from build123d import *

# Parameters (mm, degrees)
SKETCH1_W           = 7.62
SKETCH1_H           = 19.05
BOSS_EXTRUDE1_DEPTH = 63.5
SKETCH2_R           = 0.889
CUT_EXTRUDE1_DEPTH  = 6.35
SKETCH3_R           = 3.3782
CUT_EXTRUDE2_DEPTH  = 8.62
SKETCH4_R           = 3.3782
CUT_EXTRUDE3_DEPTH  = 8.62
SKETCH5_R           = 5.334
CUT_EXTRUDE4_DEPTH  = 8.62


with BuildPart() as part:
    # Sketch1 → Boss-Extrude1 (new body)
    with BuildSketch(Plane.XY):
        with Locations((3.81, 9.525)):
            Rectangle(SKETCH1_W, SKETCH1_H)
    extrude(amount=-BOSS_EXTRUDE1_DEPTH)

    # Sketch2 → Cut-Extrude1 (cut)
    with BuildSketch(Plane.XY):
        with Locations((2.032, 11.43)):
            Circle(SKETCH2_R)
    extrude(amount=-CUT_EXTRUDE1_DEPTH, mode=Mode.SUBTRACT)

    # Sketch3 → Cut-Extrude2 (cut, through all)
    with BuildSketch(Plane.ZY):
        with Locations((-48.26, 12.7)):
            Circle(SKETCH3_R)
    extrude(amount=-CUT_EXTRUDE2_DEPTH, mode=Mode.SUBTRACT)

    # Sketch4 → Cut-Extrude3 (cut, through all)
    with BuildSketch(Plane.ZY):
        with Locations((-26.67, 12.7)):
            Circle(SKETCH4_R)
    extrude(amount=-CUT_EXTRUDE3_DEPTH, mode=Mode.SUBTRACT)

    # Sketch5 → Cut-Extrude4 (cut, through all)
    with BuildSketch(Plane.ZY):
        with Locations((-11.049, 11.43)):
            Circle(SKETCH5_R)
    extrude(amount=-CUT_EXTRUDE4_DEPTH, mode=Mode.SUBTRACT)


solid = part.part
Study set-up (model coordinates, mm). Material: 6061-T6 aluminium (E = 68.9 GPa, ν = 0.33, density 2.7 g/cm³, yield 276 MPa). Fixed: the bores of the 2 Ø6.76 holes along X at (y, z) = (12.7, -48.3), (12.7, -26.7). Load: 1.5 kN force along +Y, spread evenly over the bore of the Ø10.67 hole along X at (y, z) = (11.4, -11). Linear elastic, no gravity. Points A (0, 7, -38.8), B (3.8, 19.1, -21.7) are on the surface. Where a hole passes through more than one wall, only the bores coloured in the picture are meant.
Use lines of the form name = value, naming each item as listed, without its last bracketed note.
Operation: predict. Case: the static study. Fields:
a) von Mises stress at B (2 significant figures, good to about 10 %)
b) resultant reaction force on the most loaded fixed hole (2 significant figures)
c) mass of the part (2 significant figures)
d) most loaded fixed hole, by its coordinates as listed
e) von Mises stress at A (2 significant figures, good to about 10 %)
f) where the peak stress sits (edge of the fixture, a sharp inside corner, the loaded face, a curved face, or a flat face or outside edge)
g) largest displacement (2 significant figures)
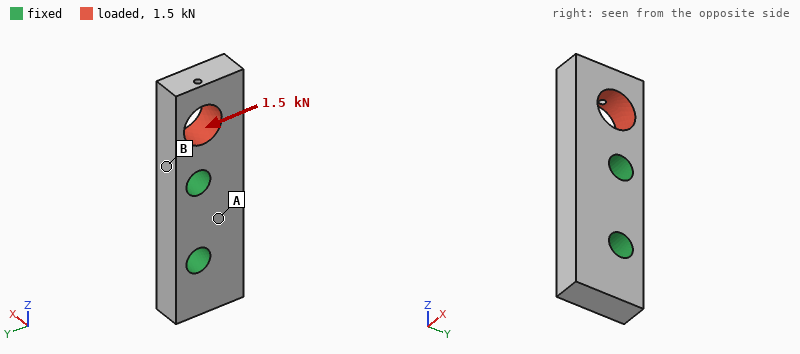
von Mises stress at B = 47 MPa
resultant reaction force on the most loaded fixed hole = 2.0 kN
mass of the part = 22 g
most loaded fixed hole, by its coordinates as listed = (12.7, -26.7)
von Mises stress at A = 11 MPa
where the peak stress sits = edge of the fixture
largest displacement = 46 µm
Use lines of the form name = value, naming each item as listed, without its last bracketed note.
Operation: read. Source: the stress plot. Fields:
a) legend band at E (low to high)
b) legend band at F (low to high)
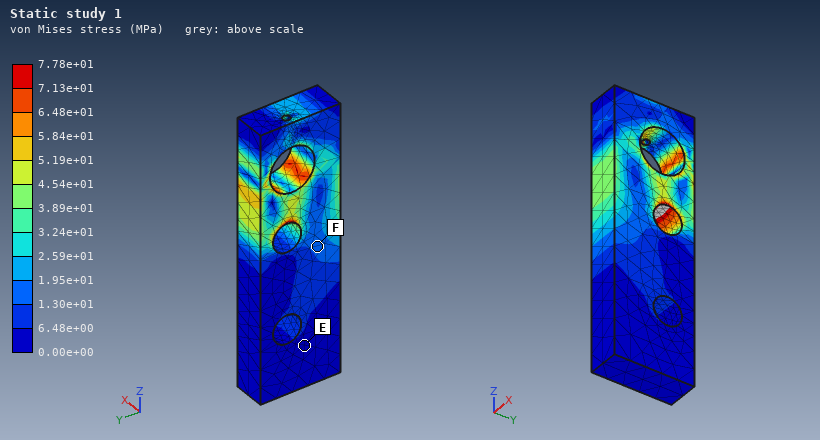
legend band at E = 0.00e+00 to 6.48e+00 MPa
legend band at F = 1.30e+01 to 1.95e+01 MPa
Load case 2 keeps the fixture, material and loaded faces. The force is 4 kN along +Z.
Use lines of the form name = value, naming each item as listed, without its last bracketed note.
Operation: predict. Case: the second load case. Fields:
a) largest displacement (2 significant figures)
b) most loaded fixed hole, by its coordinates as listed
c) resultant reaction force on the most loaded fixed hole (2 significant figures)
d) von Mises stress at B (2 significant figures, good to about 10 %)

largest displacement = 20 µm
most loaded fixed hole, by its coordinates as listed = (12.7, -26.7)
resultant reaction force on the most loaded fixed hole = 3.6 kN
von Mises stress at B = 46 MPa
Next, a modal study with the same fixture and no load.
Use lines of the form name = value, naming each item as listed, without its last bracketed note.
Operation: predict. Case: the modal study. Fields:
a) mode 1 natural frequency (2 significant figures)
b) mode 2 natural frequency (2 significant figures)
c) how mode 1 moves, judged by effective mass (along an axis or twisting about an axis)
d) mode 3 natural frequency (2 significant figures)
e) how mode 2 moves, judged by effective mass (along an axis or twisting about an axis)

mode 1 natural frequency = 8400 Hz
mode 2 natural frequency = 13 kHz
how mode 1 moves, judged by effective mass = along X
mode 3 natural frequency = 17 kHz
how mode 2 moves, judged by effective mass = along Y
